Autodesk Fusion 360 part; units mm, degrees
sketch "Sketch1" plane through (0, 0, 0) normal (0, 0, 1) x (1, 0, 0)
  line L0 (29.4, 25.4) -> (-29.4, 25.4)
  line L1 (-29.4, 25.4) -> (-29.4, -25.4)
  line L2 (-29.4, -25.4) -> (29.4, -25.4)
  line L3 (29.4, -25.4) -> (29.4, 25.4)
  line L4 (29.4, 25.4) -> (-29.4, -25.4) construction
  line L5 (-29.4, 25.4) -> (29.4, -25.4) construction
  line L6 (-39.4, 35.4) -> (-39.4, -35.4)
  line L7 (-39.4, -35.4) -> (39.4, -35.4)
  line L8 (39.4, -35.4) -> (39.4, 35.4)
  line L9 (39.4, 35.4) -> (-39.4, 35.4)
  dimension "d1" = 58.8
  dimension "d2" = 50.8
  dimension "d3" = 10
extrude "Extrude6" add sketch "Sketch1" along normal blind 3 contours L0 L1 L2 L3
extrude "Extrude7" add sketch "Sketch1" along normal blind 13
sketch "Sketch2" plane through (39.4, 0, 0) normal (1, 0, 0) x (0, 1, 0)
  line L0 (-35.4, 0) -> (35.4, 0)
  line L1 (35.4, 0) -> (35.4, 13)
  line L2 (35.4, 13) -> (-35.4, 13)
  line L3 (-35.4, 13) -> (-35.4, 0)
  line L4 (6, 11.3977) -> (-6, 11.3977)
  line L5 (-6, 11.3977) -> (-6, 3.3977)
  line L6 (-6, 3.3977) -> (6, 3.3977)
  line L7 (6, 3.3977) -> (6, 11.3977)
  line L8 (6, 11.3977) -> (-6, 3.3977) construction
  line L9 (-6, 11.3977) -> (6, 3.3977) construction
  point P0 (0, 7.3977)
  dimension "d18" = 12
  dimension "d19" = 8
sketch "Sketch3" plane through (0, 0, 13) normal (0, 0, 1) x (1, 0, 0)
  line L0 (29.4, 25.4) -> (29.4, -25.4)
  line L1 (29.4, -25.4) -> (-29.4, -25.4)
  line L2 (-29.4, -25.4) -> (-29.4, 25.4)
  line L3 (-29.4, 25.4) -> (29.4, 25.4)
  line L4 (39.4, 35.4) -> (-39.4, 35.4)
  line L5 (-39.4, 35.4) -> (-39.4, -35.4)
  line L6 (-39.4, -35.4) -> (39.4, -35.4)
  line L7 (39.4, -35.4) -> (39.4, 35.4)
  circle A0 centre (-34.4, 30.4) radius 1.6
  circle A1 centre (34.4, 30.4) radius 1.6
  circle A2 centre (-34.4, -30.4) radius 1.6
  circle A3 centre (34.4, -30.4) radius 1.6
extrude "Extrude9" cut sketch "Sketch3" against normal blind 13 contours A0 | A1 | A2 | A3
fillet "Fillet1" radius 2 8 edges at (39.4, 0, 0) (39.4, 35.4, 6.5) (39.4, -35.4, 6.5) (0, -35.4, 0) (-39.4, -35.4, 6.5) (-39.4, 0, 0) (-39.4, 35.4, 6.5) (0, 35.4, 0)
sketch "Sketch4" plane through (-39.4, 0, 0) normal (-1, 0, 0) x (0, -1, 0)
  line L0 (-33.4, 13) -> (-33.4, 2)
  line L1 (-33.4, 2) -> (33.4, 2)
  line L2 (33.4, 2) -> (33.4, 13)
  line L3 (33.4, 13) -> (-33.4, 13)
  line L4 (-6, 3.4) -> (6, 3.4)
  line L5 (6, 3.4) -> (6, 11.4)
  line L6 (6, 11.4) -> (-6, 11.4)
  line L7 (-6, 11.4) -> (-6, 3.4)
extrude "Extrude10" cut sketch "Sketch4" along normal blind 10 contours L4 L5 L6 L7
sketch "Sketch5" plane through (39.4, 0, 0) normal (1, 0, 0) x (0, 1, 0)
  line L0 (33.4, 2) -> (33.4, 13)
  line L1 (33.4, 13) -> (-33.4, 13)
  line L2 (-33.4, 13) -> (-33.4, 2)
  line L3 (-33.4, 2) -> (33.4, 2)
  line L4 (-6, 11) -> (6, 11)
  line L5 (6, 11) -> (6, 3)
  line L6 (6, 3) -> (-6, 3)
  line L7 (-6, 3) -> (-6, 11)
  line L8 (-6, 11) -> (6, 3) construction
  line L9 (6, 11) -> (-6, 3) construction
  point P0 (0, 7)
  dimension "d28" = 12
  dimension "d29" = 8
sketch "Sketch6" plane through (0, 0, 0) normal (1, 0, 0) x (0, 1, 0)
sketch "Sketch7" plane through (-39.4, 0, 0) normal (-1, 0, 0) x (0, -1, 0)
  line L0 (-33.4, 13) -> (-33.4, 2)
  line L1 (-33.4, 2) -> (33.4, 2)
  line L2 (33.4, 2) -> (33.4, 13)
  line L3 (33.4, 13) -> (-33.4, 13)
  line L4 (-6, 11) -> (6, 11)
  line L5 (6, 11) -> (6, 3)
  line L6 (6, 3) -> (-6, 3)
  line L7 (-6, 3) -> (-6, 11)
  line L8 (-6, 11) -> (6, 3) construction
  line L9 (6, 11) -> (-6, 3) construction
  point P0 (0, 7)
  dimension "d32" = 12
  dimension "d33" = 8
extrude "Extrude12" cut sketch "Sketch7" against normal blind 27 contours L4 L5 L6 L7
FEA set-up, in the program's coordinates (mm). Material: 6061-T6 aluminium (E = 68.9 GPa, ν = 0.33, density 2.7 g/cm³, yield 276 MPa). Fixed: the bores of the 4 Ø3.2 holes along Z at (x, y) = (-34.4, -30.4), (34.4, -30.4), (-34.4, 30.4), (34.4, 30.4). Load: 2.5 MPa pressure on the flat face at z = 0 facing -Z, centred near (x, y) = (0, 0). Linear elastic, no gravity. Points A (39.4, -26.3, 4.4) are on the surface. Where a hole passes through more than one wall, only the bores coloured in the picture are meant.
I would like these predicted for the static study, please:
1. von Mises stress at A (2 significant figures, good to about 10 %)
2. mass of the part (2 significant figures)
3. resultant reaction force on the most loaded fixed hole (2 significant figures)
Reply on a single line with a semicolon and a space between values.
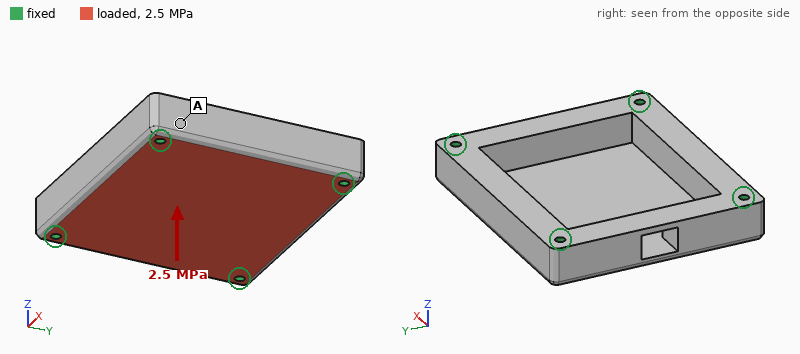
19 MPa; 110 g; 3.5 kN
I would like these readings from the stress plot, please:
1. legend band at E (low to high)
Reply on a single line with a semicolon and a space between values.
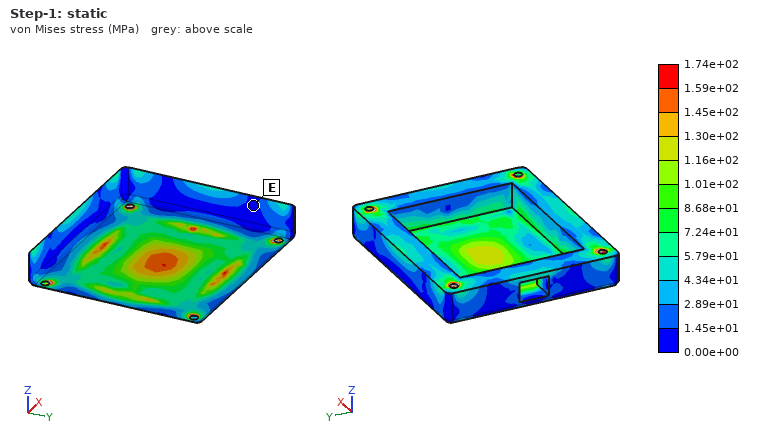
0.00e+00 to 1.45e+01 MPa
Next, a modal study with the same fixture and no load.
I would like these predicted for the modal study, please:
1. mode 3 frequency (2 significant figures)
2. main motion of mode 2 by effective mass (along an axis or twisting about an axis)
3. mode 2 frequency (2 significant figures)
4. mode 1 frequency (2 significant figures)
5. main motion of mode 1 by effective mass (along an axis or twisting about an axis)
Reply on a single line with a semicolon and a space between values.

12 kHz; twisting about X; 10 kHz; 6600 Hz; along Z
